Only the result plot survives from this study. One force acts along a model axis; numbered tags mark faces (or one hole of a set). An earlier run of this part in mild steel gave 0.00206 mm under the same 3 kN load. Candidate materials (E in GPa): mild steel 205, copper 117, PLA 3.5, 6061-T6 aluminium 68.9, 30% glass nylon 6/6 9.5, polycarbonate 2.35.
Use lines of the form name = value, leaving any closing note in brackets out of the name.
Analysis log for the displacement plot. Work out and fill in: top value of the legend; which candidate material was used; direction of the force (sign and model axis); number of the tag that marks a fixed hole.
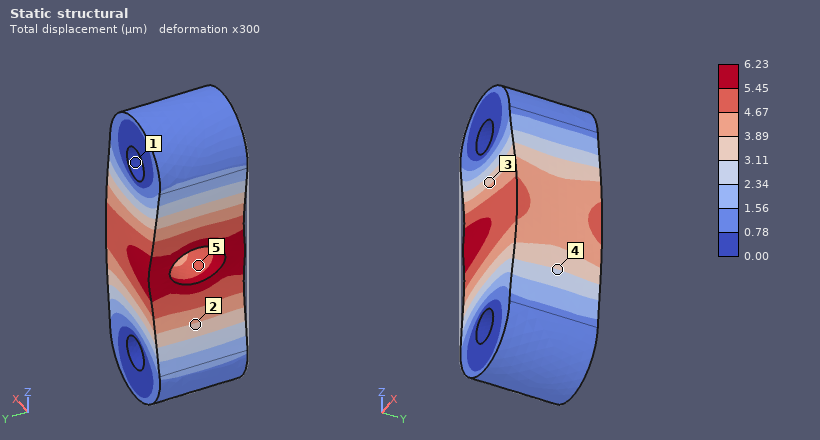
top value of the legend = 6.23 µm
which candidate material was used = 6061-T6 aluminium
direction of the force = +X
number of the tag that marks a fixed hole = 1
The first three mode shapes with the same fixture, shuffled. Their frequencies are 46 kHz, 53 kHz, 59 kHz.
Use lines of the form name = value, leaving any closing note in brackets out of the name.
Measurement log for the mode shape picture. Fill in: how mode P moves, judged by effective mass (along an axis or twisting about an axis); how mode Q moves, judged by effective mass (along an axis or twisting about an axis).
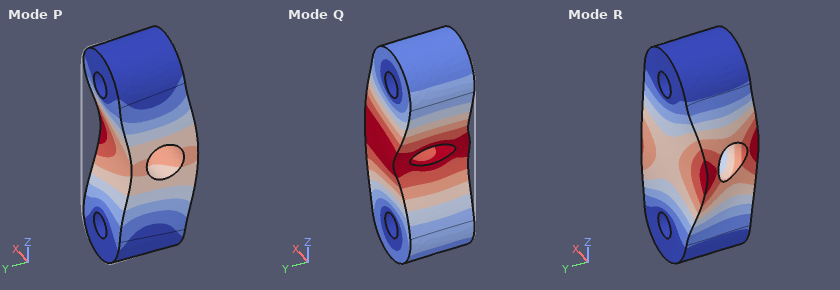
how mode P moves, judged by effective mass = along Y
how mode Q moves, judged by effective mass = along X
